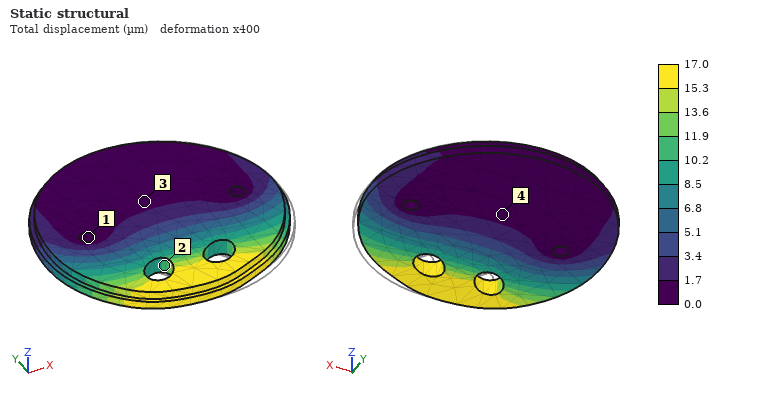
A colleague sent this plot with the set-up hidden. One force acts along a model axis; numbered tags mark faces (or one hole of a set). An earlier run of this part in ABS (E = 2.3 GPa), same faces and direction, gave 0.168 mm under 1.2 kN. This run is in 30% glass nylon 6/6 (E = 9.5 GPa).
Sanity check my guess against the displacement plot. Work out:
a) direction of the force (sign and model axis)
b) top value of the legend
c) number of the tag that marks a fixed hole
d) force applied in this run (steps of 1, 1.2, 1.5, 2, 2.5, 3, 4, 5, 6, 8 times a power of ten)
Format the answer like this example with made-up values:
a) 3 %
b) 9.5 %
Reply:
a) -X
b) 17.0 µm
c) 1
d) 500 N
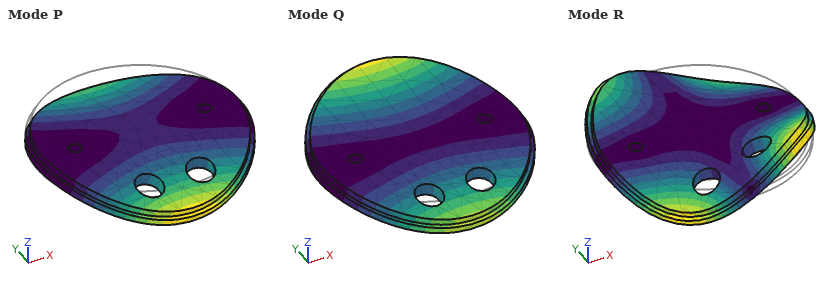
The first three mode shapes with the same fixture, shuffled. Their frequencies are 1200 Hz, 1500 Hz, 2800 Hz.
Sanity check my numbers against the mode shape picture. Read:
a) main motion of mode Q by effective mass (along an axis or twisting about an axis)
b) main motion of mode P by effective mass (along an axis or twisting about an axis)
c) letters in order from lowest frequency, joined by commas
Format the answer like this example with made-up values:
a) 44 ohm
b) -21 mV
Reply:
a) twisting about X
b) along Z
c) Q, P, R
